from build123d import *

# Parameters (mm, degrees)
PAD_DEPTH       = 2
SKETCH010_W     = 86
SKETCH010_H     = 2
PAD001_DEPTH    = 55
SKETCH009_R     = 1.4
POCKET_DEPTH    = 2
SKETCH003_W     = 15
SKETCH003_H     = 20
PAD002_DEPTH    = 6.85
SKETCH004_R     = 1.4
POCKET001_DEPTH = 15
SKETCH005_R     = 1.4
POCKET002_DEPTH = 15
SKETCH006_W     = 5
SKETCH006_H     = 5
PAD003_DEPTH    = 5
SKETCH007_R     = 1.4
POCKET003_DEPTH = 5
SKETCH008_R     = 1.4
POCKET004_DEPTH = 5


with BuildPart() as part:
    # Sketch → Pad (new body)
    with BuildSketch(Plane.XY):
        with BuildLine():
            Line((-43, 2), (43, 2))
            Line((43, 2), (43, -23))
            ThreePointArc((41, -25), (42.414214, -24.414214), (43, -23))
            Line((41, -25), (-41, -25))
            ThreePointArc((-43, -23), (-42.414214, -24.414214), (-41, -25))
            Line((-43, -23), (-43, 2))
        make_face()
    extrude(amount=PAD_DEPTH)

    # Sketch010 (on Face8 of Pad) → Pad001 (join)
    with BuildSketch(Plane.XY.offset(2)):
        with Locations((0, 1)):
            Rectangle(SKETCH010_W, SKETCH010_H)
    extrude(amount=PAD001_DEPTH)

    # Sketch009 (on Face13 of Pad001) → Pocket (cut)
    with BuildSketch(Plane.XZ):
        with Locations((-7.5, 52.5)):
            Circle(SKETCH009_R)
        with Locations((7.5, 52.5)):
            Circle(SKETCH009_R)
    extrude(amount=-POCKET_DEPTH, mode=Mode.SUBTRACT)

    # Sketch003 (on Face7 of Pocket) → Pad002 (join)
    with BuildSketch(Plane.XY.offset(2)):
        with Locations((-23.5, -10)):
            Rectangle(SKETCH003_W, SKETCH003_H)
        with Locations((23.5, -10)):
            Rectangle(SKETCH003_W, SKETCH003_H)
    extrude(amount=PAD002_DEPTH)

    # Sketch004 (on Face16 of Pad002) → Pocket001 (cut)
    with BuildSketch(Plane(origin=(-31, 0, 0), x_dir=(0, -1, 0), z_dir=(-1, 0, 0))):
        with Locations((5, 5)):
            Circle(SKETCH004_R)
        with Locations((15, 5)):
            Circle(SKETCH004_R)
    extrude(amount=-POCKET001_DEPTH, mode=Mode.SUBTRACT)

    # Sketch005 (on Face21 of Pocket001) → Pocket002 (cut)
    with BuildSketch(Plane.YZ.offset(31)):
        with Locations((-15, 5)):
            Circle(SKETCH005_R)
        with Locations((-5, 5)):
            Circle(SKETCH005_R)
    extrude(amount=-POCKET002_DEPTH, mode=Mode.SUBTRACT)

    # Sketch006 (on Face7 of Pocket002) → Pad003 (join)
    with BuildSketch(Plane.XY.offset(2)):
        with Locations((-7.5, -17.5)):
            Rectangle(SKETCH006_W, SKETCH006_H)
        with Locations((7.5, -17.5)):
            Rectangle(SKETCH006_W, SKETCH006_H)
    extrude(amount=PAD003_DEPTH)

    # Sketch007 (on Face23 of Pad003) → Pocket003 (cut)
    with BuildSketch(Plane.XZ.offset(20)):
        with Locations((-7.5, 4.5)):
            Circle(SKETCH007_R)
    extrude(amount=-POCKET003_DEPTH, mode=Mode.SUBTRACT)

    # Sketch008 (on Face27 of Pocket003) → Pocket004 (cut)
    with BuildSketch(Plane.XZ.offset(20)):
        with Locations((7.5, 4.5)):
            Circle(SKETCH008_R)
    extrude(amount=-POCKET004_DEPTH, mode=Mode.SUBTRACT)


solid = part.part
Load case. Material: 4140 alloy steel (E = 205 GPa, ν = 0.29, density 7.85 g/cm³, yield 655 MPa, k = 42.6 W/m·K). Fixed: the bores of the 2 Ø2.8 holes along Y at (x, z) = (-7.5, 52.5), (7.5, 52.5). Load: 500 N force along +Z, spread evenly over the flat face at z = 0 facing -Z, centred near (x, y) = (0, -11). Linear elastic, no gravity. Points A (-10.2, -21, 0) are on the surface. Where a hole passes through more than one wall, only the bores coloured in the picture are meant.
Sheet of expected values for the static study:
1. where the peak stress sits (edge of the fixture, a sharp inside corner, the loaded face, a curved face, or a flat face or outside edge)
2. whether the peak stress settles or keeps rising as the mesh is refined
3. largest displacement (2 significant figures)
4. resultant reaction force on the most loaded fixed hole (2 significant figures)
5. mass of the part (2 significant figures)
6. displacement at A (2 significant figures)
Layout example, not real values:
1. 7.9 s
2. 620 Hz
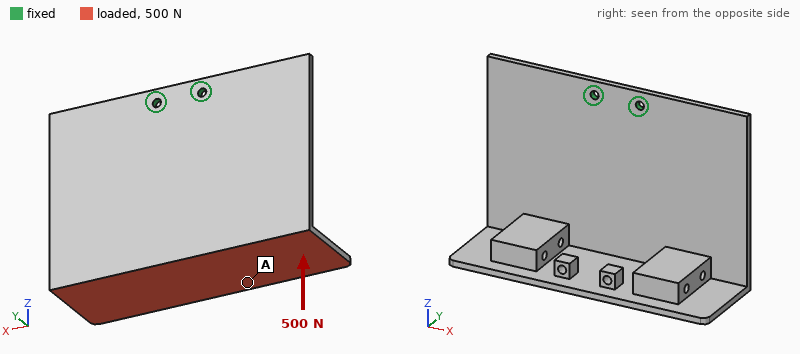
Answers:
1. edge of the fixture
2. keeps rising
3. 1.2 mm
4. 250 N
5. 140 g
6. 1.2 mm
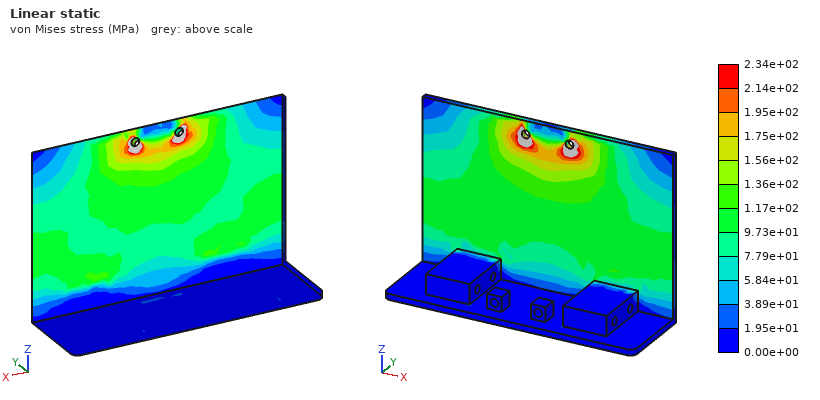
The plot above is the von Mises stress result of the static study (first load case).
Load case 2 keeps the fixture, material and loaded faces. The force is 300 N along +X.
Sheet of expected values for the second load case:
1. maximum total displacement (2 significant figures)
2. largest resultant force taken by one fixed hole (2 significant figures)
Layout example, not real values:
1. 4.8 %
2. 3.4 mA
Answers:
1. 0.44 mm
2. 930 N
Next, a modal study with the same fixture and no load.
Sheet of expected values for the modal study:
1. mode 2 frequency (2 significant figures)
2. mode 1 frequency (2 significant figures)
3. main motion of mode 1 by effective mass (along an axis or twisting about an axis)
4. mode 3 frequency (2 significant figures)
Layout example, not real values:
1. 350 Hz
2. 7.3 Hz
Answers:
1. 380 Hz
2. 220 Hz
3. along Y
4. 1200 Hz
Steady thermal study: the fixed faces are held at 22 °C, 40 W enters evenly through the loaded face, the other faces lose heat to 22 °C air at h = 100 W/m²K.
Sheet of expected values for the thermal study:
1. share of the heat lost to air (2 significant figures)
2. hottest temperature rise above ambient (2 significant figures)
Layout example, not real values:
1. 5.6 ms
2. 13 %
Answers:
1. 96 %
2. 65 K
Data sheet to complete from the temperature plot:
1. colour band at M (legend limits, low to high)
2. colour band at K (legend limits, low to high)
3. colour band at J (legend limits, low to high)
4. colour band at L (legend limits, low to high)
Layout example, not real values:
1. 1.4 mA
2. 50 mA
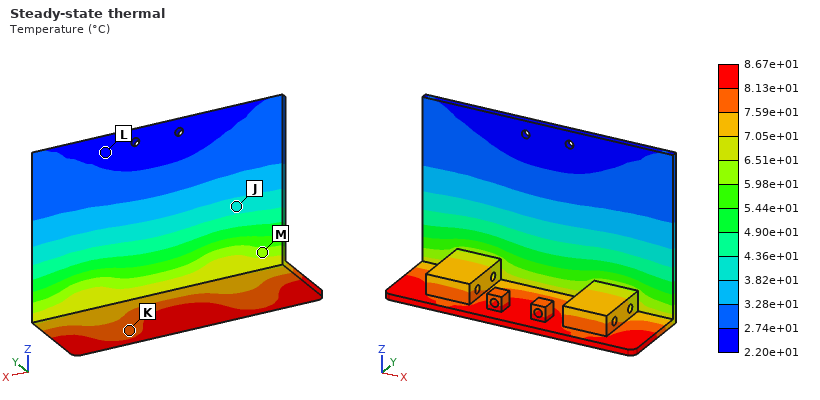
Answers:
1. 5.98e+01 to 6.51e+01 °C
2. 7.59e+01 to 8.13e+01 °C
3. 3.82e+01 to 4.36e+01 °C
4. 2.20e+01 to 2.74e+01 °C
